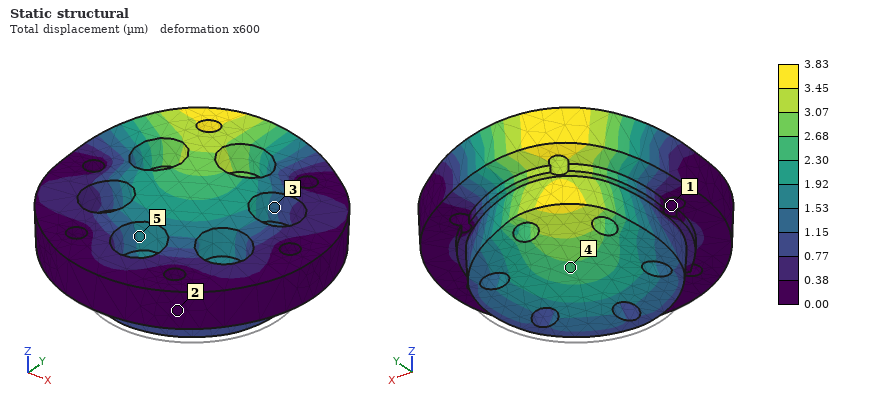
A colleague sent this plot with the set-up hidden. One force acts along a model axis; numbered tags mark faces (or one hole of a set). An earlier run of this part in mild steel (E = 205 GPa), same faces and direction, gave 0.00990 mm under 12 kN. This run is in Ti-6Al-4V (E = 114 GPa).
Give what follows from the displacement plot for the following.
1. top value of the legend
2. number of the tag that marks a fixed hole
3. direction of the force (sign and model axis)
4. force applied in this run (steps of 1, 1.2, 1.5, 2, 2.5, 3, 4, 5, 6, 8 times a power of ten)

3.83 µm
1
+Z
2.5 kN
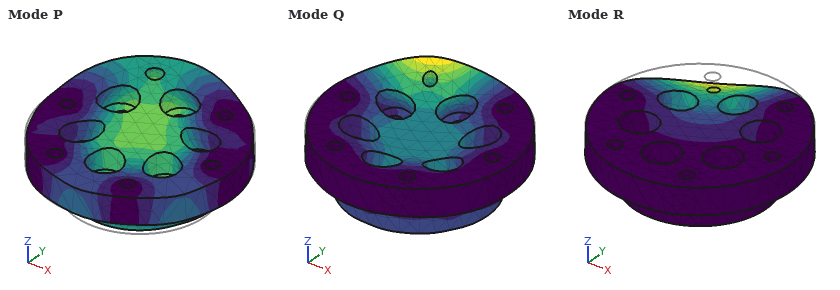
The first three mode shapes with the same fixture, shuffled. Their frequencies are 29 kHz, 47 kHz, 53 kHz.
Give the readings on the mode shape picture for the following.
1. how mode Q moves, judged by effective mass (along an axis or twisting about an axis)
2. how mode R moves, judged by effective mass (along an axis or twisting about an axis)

along Z
along Z
